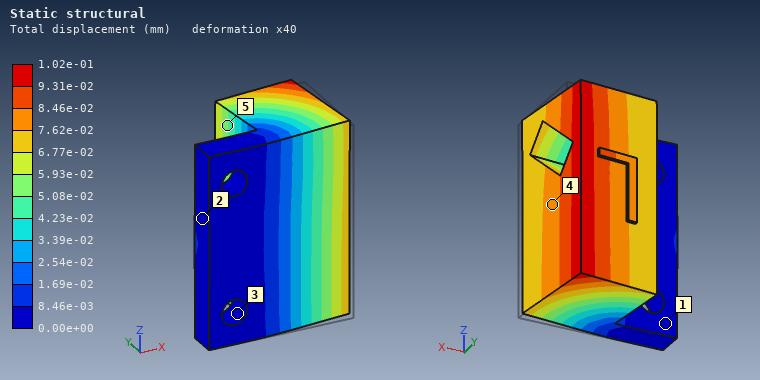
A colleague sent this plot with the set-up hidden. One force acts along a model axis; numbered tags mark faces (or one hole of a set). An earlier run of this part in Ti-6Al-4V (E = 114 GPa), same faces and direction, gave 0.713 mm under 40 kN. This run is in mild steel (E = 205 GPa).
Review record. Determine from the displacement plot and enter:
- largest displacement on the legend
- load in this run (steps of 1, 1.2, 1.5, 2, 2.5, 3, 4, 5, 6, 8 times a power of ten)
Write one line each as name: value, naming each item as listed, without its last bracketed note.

largest displacement on the legend: 1.02e-01 mm
load in this run: 10 kN
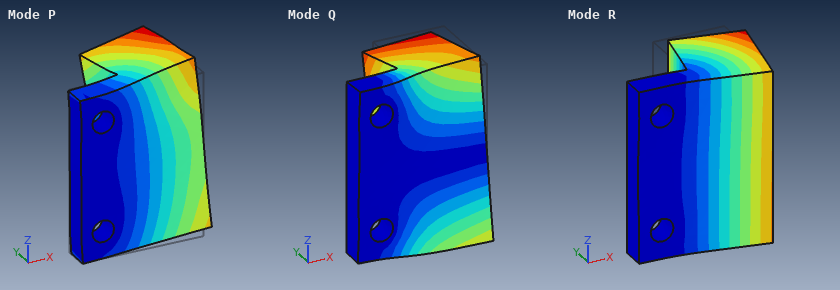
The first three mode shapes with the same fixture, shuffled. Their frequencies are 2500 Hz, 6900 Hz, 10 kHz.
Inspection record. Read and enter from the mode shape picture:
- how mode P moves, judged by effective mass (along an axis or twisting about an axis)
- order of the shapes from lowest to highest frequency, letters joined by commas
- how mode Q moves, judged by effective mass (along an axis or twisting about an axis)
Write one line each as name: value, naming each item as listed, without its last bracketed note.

how mode P moves, judged by effective mass: along Z
order of the shapes from lowest to highest frequency, letters joined by commas: R, Q, P
how mode Q moves, judged by effective mass: along Z
